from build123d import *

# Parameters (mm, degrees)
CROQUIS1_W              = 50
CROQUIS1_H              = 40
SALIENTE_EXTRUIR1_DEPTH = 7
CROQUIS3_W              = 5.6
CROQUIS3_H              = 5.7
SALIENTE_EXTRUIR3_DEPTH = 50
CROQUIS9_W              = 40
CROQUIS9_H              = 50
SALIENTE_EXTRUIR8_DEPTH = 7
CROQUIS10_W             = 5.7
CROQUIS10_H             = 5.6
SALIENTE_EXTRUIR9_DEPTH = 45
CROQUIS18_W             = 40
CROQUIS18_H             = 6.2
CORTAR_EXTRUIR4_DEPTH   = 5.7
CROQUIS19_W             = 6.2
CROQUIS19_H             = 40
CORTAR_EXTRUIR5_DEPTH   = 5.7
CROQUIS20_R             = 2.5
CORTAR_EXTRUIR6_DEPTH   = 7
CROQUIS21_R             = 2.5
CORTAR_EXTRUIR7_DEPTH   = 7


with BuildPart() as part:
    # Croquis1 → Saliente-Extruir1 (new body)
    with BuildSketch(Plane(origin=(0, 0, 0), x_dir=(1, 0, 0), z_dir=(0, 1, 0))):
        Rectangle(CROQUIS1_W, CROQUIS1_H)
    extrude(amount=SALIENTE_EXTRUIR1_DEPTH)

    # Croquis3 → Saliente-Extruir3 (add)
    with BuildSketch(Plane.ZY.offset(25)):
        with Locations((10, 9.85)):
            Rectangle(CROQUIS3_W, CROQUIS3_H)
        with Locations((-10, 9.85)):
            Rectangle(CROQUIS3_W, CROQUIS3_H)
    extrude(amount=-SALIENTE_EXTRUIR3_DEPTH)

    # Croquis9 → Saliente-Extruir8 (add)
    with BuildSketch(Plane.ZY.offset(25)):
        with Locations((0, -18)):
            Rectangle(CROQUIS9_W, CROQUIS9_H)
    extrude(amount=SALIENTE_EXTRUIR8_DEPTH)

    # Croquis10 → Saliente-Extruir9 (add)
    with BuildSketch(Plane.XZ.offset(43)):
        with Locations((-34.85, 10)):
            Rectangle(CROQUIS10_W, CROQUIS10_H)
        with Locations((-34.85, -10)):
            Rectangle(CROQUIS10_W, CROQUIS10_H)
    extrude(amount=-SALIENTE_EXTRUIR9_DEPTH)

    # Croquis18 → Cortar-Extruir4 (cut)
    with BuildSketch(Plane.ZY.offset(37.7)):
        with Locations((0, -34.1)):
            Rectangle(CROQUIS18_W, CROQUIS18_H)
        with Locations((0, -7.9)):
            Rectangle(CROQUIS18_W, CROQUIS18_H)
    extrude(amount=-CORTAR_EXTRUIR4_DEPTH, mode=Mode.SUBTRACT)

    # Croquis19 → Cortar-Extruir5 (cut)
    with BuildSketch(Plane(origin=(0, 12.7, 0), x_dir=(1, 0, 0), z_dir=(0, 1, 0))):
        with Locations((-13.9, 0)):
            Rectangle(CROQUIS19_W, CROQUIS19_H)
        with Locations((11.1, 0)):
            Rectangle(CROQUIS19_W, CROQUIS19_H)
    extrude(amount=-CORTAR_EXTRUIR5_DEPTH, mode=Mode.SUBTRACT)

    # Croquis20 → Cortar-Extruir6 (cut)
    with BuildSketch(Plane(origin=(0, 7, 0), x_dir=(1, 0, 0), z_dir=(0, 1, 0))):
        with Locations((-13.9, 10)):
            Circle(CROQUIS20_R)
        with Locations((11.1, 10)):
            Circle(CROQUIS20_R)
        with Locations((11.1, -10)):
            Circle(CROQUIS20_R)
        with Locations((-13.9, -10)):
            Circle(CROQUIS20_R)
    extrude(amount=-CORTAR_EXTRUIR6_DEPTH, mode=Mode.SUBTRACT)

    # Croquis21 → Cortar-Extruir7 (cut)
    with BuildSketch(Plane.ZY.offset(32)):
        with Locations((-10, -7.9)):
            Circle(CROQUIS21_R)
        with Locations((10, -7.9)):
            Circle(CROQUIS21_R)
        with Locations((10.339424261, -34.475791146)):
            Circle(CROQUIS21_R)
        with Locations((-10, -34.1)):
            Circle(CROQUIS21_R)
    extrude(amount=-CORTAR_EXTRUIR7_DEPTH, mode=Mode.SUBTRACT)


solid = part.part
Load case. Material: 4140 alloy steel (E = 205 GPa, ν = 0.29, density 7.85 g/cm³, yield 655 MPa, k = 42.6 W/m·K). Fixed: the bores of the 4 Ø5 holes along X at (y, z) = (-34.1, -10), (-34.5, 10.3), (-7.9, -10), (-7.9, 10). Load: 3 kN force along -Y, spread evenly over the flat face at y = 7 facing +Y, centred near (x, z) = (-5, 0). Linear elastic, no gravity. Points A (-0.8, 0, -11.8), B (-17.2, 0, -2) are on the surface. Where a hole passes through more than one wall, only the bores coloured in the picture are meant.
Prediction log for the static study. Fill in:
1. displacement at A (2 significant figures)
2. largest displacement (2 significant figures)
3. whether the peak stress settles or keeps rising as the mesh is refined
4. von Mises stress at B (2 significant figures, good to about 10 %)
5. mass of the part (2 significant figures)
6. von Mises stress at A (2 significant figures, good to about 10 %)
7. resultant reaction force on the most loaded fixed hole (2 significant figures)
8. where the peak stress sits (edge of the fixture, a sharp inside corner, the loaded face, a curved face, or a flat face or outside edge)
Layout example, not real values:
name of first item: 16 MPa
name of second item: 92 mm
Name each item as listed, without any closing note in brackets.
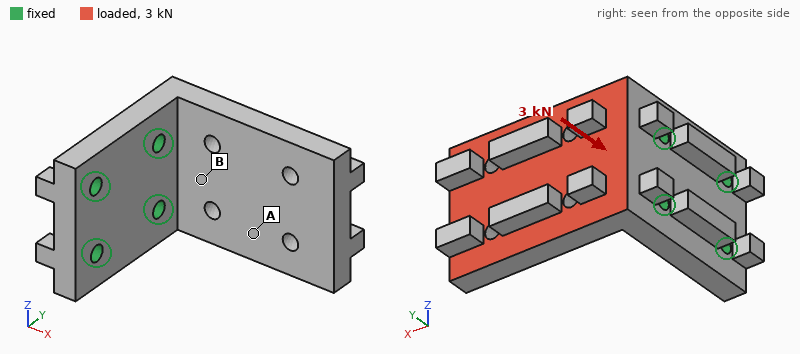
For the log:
displacement at A: 0.15 mm
largest displacement: 0.35 mm
whether the peak stress settles or keeps rising as the mesh is refined: keeps rising
von Mises stress at B: 140 MPa
mass of the part: 250 g
von Mises stress at A: 34 MPa
resultant reaction force on the most loaded fixed hole: 1.5 kN
where the peak stress sits: edge of the fixture
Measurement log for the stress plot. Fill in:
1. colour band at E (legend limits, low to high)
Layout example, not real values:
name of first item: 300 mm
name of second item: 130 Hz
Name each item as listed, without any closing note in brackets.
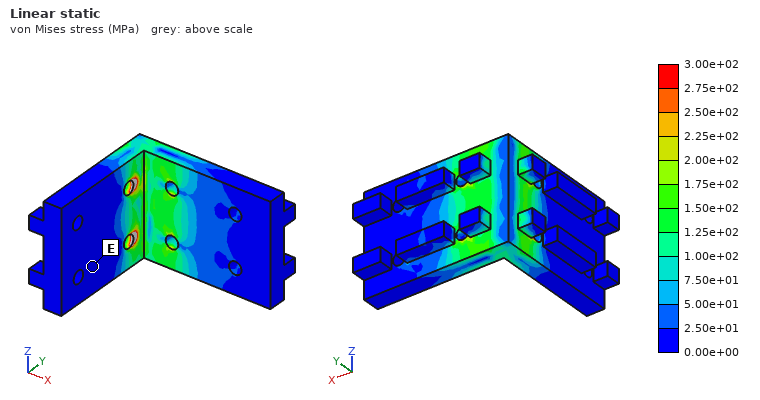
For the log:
colour band at E: 0.00e+00 to 2.50e+01 MPa
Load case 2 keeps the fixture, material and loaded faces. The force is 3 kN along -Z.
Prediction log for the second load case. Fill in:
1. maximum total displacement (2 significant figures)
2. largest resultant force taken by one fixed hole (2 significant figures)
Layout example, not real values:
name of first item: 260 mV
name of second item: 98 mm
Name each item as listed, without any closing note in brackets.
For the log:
maximum total displacement: 47 µm
largest resultant force taken by one fixed hole: 3.5 kN
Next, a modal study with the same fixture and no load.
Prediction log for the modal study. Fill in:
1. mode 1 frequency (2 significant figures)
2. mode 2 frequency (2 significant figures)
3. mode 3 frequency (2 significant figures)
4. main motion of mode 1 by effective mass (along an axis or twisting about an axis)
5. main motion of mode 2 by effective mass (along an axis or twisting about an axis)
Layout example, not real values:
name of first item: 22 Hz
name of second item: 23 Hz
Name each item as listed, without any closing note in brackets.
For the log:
mode 1 frequency: 1500 Hz
mode 2 frequency: 3700 Hz
mode 3 frequency: 5400 Hz
main motion of mode 1 by effective mass: along Y
main motion of mode 2 by effective mass: along Z
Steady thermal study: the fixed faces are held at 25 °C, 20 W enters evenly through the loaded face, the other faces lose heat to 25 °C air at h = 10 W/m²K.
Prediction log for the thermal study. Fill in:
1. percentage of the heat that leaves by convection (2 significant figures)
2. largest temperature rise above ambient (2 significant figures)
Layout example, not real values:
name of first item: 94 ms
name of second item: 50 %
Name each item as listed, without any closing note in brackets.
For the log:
percentage of the heat that leaves by convection: 10 %
largest temperature rise above ambient: 50 K
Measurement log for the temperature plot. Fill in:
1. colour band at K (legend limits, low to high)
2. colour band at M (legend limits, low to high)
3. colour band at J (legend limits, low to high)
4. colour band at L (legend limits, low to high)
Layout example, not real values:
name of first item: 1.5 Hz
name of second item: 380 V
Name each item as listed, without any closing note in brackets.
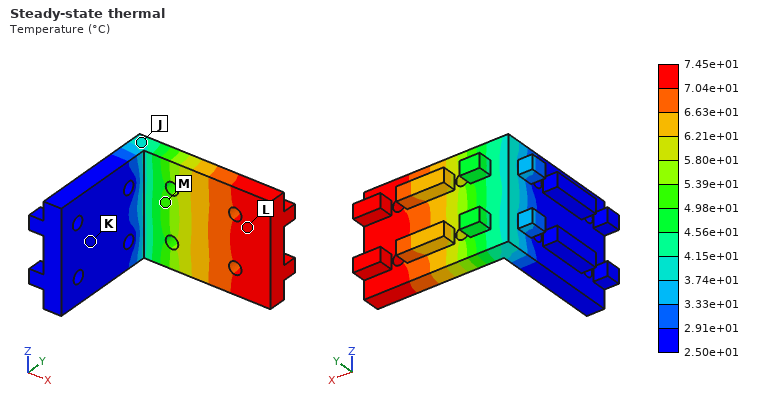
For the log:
colour band at K: 2.50e+01 to 2.91e+01 °C
colour band at M: 4.98e+01 to 5.39e+01 °C
colour band at J: 3.74e+01 to 4.15e+01 °C
colour band at L: 7.04e+01 to 7.45e+01 °C
